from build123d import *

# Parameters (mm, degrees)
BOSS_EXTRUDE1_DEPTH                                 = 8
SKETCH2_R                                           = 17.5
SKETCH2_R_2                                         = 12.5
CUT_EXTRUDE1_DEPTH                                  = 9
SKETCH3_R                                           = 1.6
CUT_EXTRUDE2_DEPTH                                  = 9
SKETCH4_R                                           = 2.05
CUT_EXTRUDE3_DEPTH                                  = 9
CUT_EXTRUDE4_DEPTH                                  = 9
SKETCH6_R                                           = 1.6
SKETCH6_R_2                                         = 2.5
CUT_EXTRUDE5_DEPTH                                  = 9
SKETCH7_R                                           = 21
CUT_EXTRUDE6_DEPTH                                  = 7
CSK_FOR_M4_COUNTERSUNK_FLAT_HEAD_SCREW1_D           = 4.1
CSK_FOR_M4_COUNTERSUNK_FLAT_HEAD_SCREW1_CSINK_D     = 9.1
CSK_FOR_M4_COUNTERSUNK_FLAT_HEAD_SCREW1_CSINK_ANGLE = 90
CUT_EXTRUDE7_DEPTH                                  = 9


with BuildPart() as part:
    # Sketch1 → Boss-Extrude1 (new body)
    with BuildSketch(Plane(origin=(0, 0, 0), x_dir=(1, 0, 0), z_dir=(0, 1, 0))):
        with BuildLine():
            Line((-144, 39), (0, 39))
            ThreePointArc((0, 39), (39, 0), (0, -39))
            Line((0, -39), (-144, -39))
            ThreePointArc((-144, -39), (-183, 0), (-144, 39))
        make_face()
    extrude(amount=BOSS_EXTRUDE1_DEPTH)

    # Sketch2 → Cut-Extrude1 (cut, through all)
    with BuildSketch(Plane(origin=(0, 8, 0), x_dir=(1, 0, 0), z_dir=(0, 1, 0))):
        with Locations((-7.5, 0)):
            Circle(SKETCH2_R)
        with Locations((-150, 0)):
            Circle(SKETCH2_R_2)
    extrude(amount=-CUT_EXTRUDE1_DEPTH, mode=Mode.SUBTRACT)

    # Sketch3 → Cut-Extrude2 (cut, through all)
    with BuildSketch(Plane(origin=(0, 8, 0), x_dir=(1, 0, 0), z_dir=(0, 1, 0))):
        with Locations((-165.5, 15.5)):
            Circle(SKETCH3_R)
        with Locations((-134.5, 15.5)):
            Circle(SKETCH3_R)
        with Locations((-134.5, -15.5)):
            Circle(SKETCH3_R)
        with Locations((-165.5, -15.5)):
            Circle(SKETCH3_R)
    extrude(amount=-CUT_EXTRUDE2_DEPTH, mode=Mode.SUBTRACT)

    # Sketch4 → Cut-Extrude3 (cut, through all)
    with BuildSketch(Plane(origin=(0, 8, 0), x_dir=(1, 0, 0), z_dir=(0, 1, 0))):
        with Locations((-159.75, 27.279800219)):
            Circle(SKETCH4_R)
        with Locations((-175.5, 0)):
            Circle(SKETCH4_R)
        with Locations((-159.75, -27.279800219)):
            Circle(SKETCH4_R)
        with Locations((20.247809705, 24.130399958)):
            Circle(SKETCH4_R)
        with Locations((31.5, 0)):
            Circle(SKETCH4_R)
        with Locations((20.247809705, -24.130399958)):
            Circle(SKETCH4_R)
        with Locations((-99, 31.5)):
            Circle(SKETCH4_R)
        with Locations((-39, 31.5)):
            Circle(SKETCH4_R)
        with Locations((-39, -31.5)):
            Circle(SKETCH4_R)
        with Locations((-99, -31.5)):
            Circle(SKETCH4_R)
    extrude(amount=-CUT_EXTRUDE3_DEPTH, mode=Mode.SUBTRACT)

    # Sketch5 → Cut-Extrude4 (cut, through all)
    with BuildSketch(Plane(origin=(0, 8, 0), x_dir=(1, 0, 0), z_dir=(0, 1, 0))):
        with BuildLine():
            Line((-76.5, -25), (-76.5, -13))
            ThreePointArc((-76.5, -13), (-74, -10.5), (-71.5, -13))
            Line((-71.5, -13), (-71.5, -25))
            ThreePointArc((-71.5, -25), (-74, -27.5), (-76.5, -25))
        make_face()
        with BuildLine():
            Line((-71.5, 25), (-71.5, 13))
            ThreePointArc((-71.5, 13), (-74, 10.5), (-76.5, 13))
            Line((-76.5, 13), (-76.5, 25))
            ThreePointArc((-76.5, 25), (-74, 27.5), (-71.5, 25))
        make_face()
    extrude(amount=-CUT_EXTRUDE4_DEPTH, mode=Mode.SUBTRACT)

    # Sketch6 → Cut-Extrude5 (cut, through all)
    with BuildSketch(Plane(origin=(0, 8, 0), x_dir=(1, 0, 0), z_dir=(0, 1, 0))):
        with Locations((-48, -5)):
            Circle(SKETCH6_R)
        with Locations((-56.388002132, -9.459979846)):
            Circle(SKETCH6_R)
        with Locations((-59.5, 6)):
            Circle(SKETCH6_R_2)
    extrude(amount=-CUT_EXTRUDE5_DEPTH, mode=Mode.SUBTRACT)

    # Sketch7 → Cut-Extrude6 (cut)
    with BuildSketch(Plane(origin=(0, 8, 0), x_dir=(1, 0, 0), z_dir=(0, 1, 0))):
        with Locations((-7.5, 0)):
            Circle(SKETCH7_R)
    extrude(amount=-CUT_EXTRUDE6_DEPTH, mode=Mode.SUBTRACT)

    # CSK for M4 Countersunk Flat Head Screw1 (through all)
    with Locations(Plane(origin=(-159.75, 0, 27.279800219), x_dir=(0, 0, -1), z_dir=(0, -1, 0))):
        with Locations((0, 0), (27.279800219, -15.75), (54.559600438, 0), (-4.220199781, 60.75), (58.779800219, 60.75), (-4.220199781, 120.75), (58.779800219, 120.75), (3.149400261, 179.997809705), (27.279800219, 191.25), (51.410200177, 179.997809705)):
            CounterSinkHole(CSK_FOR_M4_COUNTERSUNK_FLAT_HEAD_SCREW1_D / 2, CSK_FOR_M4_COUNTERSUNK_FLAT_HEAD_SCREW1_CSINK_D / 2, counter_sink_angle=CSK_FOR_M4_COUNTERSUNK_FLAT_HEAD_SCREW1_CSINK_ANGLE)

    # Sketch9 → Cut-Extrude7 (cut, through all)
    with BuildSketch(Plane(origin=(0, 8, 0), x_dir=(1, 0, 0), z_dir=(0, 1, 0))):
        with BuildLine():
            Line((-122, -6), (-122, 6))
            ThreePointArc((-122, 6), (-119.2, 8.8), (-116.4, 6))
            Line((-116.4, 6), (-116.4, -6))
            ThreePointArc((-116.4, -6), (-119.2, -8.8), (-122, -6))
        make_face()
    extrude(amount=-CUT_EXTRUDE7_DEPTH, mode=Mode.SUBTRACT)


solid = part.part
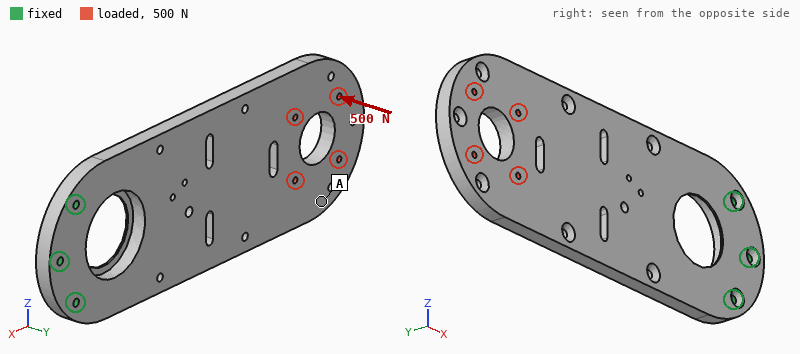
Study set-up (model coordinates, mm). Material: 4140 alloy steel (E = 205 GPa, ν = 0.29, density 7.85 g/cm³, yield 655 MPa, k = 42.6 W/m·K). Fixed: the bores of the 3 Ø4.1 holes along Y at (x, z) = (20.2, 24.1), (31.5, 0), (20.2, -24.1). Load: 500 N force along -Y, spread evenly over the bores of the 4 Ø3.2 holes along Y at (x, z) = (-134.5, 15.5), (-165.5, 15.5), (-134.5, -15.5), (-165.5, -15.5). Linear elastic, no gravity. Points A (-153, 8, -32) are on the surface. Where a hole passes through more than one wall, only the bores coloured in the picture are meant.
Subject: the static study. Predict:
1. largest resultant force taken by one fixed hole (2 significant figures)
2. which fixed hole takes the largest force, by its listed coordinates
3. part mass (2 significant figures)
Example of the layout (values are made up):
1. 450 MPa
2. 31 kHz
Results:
1. 1.4 kN
2. (31.5, 0)
3. 860 g
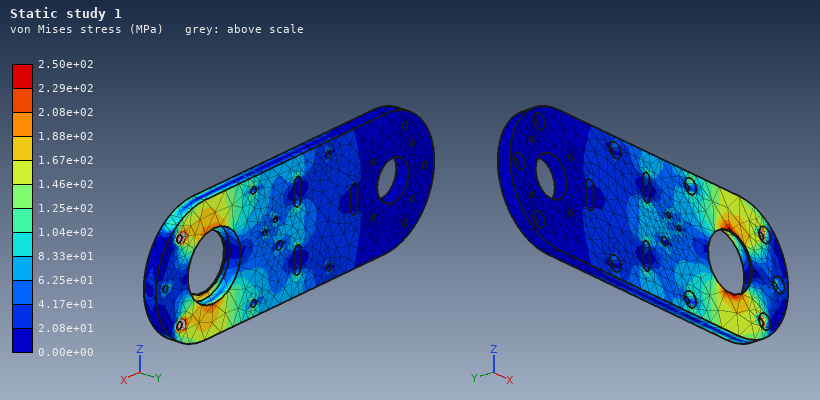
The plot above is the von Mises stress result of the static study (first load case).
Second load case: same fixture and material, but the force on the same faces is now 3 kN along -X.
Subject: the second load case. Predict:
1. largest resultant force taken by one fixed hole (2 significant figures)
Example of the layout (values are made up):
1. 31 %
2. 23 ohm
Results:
1. 1.5 kN
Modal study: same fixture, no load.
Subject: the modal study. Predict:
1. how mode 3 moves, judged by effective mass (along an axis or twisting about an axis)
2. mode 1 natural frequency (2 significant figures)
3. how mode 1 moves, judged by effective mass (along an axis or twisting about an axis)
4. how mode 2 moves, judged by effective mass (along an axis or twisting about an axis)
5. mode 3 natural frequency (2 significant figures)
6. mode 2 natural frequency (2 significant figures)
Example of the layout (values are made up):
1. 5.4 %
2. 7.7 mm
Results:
1. along Y
2. 140 Hz
3. along Y
4. twisting about X
5. 920 Hz
6. 790 Hz
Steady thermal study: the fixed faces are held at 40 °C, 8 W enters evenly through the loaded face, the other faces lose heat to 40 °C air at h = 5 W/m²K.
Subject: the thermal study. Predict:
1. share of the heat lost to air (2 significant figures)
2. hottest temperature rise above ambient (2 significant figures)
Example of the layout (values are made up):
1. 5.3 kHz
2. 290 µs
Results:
1. 52 %
2. 46 K
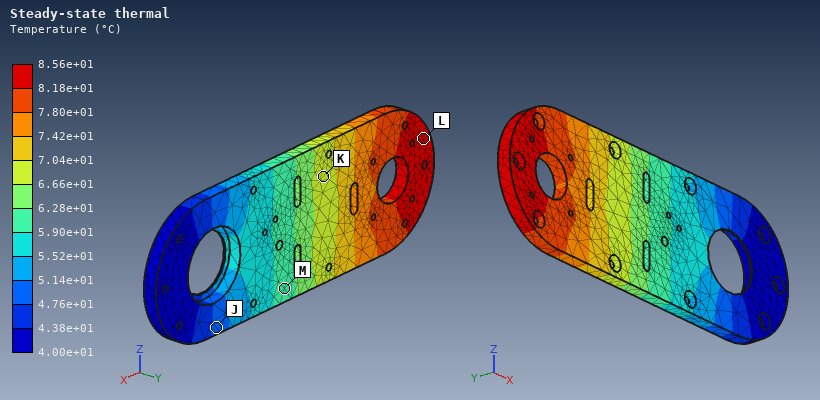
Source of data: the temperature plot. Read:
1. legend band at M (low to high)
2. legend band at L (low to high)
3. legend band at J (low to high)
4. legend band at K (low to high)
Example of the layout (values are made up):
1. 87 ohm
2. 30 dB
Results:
1. 5.90e+01 to 6.28e+01 °C
2. 8.18e+01 to 8.56e+01 °C
3. 4.76e+01 to 5.14e+01 °C
4. 6.66e+01 to 7.04e+01 °C
